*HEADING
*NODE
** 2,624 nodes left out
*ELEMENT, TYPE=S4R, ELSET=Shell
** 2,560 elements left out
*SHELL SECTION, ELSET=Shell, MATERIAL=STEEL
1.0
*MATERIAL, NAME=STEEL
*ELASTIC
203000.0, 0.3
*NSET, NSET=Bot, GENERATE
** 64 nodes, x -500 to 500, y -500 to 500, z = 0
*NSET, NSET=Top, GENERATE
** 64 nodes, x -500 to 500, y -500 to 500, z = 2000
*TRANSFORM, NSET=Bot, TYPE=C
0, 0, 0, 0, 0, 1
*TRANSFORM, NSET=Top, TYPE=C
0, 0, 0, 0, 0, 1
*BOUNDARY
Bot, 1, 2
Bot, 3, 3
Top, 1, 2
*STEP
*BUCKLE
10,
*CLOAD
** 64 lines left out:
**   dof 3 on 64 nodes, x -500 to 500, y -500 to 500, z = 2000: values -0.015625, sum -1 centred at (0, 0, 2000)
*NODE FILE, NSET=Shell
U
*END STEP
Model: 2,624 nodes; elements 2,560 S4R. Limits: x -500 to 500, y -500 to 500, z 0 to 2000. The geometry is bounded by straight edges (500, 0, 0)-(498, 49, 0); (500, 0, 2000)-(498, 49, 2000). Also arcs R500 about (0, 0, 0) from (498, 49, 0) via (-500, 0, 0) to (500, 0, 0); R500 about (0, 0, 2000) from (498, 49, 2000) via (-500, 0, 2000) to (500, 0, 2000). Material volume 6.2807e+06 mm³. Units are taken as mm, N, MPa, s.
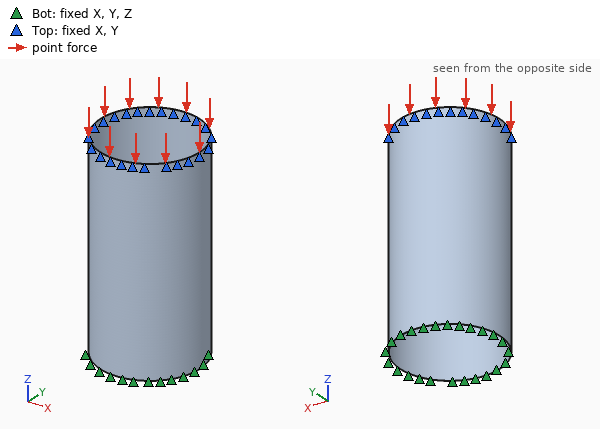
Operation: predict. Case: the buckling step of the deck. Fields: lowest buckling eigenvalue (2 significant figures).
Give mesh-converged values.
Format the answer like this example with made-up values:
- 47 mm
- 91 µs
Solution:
- 7.8e+05
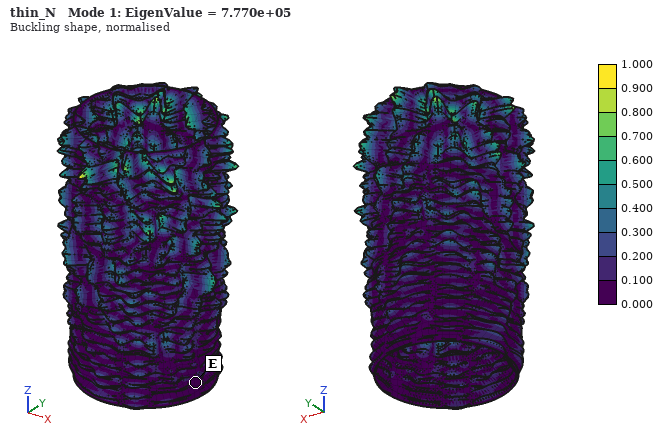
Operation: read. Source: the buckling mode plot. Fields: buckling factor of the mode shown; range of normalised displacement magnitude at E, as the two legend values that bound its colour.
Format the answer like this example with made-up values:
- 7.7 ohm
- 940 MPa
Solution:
- 7.770e+05
- 0.000 to 0.100
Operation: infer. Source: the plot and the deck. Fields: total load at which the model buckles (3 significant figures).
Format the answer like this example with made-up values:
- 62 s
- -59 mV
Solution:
- 7.77e+05 N
